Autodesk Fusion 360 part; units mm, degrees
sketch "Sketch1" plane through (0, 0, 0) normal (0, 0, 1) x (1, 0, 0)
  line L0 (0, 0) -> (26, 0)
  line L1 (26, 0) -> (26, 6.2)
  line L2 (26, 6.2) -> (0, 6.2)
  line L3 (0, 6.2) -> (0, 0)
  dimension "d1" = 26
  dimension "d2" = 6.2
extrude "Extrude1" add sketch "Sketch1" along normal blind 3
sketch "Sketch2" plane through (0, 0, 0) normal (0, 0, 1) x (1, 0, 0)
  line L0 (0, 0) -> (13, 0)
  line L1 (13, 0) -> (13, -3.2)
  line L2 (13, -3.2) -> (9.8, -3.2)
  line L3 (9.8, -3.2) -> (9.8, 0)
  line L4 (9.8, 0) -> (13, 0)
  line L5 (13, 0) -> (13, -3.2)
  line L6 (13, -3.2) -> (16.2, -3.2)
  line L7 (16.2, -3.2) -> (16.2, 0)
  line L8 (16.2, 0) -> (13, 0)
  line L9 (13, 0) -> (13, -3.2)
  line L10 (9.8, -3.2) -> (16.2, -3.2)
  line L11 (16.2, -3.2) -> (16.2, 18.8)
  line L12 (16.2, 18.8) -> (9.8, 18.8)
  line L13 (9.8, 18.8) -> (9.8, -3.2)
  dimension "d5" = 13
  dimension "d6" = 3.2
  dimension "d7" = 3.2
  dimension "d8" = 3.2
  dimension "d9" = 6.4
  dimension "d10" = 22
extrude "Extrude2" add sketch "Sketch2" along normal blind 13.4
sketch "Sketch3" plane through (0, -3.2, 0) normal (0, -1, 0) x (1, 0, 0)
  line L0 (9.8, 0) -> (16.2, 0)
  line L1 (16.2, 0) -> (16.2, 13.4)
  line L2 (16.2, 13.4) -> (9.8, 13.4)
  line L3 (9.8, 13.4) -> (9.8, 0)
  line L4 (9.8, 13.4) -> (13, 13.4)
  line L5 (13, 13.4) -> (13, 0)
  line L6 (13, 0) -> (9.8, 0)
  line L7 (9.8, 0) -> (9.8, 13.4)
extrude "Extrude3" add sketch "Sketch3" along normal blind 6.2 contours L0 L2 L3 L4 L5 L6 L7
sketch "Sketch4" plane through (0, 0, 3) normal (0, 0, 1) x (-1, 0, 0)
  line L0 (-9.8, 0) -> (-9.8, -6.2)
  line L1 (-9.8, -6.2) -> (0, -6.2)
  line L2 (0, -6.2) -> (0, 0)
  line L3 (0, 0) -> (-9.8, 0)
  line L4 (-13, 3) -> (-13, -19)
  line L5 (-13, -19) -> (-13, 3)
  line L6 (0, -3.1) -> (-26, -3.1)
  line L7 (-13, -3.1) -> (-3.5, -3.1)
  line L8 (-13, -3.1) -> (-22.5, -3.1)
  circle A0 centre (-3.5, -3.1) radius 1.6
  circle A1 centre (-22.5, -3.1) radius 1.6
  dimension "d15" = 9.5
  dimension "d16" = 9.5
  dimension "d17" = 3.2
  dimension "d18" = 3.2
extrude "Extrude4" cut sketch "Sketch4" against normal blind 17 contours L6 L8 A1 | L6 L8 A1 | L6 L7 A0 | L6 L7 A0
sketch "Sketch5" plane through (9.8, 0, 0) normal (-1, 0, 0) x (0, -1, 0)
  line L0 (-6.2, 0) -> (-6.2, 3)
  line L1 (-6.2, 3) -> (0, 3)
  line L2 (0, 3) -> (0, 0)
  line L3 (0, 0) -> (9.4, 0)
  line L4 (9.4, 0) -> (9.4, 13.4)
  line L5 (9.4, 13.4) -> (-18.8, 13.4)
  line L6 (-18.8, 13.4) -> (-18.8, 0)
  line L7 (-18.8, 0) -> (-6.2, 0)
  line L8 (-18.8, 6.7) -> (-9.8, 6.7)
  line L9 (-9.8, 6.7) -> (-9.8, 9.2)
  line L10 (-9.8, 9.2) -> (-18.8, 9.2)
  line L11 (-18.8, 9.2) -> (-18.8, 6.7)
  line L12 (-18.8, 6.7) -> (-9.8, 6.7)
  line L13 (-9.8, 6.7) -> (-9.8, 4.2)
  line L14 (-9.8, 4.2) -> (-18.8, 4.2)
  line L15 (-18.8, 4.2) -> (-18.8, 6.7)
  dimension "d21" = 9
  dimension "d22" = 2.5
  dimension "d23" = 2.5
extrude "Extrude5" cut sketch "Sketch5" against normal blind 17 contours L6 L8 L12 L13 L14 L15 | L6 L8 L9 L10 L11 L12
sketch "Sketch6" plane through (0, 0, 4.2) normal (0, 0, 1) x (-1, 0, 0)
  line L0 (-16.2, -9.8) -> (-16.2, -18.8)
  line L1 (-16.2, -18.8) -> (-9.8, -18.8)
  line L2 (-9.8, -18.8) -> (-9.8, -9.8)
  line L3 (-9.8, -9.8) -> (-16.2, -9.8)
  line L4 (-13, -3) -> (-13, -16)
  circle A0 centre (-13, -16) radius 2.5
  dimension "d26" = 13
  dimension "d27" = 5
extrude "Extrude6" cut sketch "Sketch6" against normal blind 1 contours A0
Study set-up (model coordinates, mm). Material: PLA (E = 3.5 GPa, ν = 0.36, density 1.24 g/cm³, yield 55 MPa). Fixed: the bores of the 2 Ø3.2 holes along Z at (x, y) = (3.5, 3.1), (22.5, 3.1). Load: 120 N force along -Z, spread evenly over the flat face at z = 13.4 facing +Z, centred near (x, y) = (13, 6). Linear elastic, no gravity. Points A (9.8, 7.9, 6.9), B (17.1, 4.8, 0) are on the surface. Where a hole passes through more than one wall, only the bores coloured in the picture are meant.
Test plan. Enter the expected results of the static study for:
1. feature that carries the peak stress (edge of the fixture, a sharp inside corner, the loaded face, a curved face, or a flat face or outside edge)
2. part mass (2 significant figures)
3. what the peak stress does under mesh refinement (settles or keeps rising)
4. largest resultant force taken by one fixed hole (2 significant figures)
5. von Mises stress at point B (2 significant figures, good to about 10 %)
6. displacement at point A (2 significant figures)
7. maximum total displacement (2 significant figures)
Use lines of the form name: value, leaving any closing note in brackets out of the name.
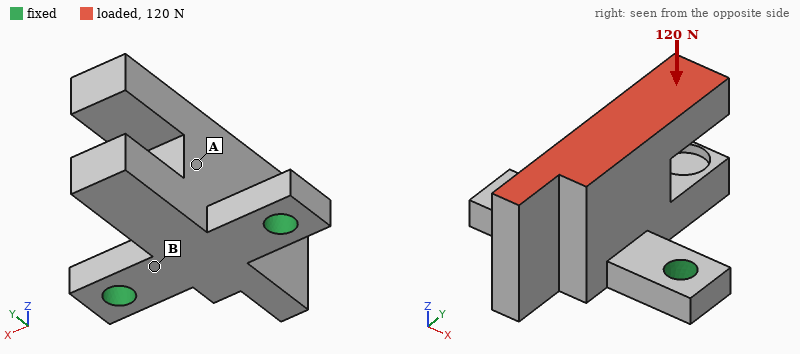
feature that carries the peak stress: edge of the fixture
part mass: 2.7 g
what the peak stress does under mesh refinement: keeps rising
largest resultant force taken by one fixed hole: 65 N
von Mises stress at point B: 17 MPa
displacement at point A: 0.17 mm
maximum total displacement: 0.48 mm
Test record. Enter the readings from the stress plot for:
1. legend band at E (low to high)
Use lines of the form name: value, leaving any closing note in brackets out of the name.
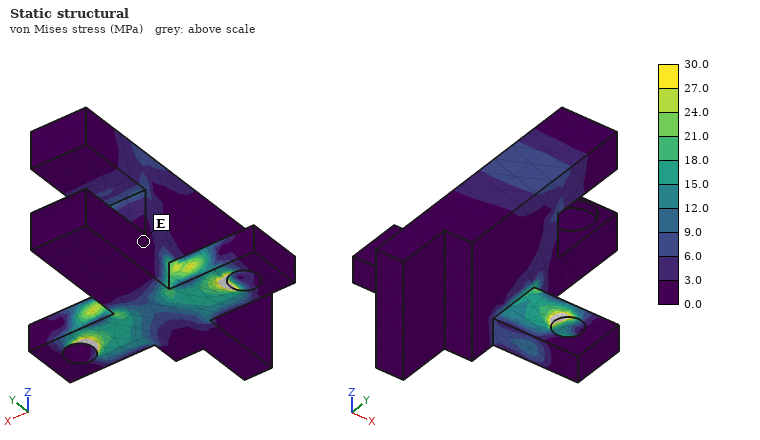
legend band at E: 0.0 to 3.0 MPa
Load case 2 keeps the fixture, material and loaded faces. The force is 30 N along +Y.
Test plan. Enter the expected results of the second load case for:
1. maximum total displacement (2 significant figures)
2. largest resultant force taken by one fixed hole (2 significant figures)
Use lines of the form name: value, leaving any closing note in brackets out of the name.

maximum total displacement: 0.39 mm
largest resultant force taken by one fixed hole: 15 N
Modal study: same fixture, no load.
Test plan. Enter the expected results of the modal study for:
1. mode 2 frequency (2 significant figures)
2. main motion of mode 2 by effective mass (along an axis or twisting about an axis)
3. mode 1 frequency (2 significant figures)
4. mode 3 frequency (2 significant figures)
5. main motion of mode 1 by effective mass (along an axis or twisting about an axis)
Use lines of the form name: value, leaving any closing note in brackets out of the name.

mode 2 frequency: 3900 Hz
main motion of mode 2 by effective mass: along X
mode 1 frequency: 1400 Hz
mode 3 frequency: 5100 Hz
main motion of mode 1 by effective mass: along Y
